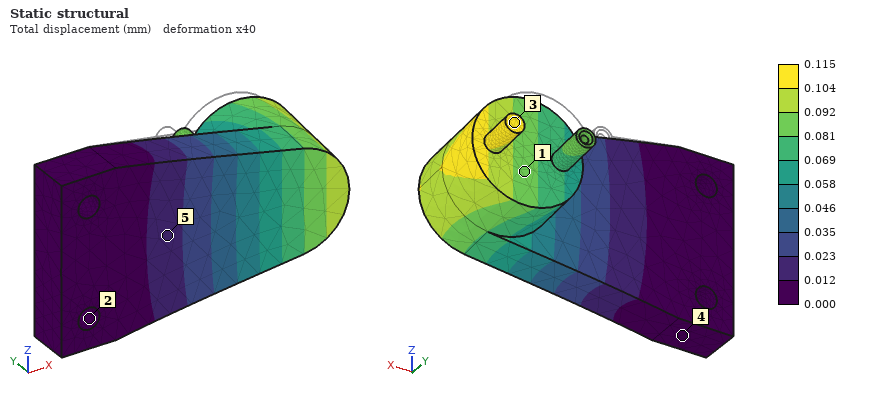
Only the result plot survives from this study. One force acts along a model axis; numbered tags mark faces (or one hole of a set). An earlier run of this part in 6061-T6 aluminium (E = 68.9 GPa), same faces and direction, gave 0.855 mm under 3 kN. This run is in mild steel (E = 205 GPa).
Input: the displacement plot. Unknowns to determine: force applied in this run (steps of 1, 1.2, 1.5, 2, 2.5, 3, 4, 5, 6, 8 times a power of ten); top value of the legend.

1.2 kN
0.115 mm
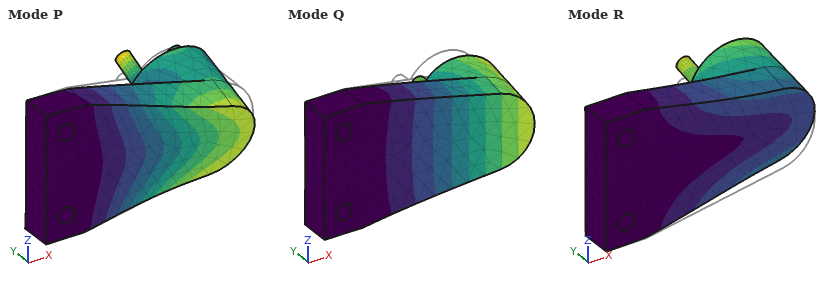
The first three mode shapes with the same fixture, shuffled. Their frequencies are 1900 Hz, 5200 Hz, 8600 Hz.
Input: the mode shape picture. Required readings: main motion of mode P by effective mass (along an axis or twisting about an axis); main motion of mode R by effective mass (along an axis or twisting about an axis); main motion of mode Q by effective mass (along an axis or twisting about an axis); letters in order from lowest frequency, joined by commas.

along Z
along Z
along Y
Q, R, P
